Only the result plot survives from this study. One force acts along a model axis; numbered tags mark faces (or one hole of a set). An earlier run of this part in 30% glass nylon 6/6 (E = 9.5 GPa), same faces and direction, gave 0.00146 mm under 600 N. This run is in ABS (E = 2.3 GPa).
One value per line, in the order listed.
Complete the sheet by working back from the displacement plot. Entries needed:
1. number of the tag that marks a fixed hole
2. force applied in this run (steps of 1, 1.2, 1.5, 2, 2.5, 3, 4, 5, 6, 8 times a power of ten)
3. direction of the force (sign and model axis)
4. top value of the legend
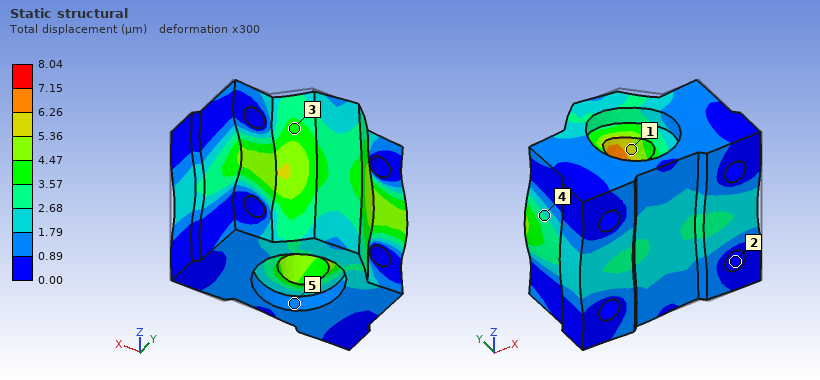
2
800 N
-X
8.04 µm
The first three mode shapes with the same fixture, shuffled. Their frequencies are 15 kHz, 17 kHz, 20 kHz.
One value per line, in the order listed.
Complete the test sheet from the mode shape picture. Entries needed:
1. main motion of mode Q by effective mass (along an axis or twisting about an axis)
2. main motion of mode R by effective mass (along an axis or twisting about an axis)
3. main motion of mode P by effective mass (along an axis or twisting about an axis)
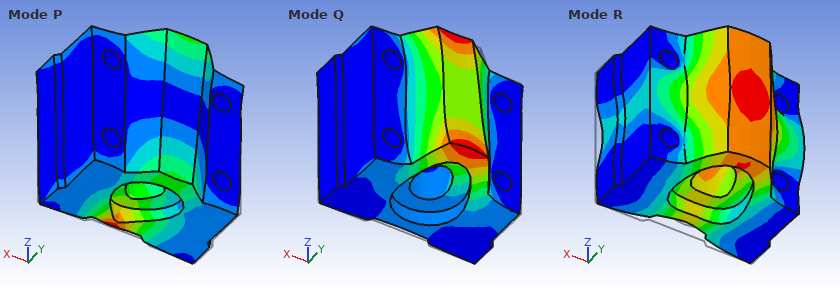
along Z
along Y
along Z
